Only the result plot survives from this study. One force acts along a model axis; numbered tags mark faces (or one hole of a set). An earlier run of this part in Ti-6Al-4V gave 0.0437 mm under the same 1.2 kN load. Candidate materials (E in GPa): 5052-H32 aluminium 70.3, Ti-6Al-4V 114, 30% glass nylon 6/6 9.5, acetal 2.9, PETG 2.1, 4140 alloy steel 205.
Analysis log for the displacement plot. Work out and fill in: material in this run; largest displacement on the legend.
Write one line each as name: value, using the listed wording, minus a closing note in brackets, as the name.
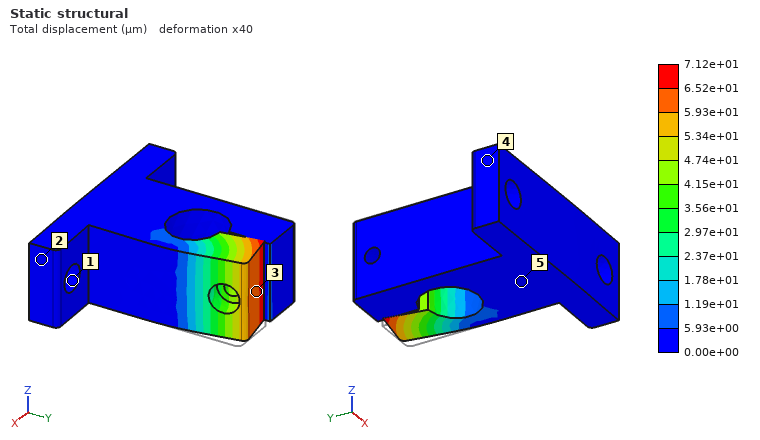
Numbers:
material in this run: 5052-H32 aluminium
largest displacement on the legend: 7.12e+01 µm
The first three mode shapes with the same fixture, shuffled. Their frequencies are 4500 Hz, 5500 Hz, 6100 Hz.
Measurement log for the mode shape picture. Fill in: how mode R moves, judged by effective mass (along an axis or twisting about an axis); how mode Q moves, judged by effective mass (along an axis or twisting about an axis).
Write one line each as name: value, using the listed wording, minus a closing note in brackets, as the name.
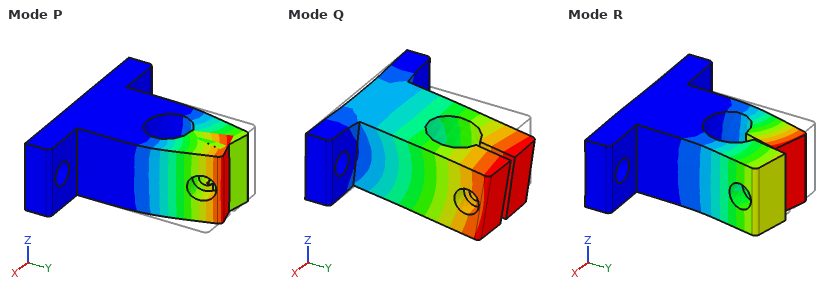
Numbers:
how mode R moves, judged by effective mass: along X
how mode Q moves, judged by effective mass: along Z
